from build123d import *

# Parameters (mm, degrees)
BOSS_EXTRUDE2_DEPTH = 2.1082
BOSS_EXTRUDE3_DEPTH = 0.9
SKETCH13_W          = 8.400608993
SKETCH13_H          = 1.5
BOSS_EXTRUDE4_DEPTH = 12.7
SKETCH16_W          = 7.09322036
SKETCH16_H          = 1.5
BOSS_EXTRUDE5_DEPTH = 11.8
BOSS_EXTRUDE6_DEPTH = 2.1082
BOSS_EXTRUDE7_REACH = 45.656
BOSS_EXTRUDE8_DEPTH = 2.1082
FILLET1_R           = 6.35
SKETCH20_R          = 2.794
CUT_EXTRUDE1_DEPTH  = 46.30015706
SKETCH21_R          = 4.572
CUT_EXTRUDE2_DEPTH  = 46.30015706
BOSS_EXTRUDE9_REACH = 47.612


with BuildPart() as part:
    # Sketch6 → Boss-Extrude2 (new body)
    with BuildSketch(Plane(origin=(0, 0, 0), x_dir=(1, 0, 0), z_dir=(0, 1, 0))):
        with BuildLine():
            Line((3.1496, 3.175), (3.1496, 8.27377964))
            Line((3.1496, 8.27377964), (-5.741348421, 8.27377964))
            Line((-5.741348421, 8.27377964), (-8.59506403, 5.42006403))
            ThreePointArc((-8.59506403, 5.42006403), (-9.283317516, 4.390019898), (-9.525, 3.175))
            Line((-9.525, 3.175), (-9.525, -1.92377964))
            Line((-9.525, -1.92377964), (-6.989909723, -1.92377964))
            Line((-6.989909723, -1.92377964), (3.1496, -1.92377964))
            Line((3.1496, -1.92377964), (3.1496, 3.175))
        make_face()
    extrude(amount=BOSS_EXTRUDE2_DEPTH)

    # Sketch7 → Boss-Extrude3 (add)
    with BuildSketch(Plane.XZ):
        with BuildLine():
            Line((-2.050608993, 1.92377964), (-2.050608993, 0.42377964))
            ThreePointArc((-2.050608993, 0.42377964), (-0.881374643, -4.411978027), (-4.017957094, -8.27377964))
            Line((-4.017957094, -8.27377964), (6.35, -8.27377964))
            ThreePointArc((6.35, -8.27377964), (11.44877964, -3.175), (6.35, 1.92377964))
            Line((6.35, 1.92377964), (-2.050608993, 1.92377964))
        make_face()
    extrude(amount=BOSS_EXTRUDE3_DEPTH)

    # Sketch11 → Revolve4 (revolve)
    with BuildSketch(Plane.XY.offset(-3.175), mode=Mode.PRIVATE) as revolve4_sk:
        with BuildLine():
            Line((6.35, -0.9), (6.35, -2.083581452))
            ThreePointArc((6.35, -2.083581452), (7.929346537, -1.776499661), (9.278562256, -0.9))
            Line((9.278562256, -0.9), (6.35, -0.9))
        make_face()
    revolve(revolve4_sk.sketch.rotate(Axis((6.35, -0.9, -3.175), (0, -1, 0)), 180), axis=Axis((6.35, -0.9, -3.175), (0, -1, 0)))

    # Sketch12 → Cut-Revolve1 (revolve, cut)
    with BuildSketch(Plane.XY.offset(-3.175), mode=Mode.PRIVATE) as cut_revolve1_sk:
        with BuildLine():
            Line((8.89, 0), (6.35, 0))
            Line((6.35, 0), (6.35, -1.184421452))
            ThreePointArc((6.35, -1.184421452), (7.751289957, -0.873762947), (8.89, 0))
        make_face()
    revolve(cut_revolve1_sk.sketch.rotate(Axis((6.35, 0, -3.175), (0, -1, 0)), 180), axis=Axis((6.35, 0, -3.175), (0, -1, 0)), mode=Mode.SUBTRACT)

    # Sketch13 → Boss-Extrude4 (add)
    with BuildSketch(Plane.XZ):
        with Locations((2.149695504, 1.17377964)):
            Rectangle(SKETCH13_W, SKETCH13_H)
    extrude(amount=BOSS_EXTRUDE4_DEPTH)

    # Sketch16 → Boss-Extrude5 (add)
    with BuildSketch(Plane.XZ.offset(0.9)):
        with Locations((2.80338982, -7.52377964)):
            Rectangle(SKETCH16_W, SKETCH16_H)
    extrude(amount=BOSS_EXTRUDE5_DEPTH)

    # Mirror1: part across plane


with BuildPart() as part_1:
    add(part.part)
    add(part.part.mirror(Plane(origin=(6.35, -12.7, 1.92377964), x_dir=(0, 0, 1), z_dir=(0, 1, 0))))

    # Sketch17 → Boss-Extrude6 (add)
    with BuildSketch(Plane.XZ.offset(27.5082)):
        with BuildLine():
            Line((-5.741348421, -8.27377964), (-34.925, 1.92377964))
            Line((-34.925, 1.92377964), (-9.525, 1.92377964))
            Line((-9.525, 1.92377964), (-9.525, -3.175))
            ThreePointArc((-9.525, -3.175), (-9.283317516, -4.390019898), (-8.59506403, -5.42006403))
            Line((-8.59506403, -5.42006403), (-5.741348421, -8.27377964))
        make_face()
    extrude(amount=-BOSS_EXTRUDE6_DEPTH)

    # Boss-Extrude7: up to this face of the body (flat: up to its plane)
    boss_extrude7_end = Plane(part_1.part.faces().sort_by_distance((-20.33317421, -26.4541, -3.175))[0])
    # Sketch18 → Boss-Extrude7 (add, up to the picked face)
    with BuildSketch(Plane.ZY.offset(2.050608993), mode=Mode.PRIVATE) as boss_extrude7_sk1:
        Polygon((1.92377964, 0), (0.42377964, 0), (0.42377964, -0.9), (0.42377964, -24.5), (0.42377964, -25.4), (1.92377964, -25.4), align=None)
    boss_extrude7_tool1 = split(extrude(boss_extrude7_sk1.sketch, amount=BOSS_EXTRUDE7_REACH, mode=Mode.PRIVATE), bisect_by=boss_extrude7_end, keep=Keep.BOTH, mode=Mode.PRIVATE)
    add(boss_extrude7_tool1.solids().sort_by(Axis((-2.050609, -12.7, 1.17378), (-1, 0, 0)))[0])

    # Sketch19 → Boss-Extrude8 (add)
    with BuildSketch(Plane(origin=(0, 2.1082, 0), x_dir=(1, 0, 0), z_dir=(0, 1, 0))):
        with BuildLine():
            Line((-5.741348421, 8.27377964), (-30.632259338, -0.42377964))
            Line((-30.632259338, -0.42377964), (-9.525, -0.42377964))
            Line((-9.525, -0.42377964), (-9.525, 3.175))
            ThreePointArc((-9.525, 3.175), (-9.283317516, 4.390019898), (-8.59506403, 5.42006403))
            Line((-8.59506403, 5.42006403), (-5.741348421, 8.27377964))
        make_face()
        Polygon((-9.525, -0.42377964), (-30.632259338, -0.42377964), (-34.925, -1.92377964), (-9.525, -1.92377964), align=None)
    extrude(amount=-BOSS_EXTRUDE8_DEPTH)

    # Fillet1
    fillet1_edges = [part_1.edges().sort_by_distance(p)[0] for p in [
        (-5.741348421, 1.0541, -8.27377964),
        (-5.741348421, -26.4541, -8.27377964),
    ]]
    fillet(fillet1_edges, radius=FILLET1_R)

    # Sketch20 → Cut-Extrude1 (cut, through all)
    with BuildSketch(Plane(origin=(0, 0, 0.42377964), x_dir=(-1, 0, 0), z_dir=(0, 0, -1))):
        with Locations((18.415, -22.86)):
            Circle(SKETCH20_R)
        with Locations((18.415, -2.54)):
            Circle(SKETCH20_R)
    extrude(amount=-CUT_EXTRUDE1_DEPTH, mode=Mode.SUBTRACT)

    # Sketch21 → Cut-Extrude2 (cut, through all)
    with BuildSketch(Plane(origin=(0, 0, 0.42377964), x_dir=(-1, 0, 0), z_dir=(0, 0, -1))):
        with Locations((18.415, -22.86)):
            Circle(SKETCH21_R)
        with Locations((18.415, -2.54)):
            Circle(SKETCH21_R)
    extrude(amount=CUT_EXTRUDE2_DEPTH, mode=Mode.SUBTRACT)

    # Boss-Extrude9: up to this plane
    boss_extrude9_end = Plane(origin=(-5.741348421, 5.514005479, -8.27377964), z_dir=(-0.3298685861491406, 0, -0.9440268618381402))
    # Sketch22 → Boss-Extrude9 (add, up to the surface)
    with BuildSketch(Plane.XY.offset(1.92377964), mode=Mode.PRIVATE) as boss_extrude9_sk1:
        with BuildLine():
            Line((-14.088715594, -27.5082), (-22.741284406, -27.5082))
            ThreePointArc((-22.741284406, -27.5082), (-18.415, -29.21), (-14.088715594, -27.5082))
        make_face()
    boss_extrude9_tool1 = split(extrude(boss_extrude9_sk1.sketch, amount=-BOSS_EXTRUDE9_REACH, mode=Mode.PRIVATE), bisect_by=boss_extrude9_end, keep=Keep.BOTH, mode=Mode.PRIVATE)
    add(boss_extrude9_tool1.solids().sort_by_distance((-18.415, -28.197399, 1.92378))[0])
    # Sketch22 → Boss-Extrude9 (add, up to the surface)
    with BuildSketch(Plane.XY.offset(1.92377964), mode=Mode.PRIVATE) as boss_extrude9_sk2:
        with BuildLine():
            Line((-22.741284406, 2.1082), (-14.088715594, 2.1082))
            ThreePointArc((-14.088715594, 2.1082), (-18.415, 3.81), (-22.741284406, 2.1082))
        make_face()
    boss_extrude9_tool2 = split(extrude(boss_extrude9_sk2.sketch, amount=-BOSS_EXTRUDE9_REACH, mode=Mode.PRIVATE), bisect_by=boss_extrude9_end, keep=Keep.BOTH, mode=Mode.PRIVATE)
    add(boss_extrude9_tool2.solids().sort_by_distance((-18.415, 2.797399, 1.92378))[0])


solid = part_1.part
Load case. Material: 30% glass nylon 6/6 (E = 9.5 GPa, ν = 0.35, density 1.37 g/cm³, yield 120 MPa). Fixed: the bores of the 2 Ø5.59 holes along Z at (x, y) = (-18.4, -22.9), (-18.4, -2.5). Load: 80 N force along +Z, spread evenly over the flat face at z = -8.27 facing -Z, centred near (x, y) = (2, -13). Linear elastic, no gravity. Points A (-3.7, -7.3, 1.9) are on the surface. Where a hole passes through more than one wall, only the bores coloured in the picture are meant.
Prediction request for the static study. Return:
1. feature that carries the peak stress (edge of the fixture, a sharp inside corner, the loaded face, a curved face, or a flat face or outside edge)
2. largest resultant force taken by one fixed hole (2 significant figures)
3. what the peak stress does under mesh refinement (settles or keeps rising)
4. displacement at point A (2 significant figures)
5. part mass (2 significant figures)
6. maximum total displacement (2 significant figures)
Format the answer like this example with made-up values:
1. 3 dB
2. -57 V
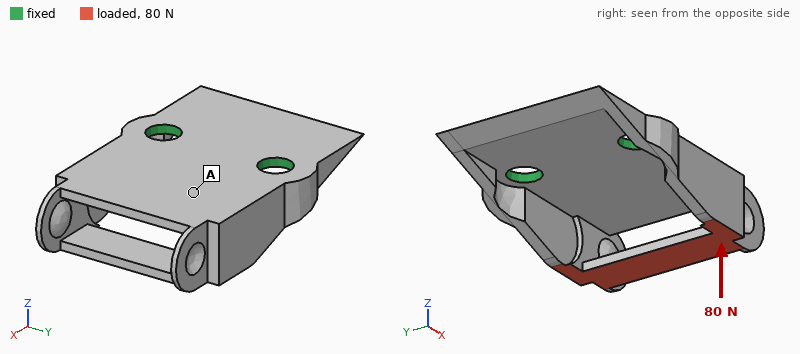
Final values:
1. edge of the fixture
2. 47 N
3. keeps rising
4. 0.23 mm
5. 4.0 g
6. 0.68 mm
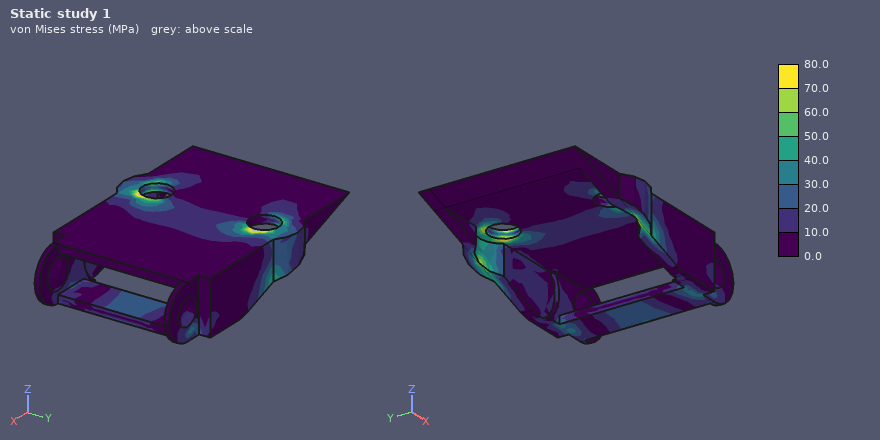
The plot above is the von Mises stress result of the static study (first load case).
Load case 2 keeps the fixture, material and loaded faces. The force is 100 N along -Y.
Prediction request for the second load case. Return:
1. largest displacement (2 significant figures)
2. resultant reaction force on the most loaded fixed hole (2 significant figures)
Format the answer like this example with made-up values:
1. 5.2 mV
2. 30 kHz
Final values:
1. 0.40 mm
2. 99 N
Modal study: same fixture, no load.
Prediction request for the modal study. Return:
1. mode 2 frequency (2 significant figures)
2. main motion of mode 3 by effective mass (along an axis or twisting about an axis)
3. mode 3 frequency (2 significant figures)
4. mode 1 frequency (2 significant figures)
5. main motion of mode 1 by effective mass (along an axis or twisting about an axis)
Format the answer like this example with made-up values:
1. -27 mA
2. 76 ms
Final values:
1. 2300 Hz
2. along Y
3. 4300 Hz
4. 1700 Hz
5. along Z
